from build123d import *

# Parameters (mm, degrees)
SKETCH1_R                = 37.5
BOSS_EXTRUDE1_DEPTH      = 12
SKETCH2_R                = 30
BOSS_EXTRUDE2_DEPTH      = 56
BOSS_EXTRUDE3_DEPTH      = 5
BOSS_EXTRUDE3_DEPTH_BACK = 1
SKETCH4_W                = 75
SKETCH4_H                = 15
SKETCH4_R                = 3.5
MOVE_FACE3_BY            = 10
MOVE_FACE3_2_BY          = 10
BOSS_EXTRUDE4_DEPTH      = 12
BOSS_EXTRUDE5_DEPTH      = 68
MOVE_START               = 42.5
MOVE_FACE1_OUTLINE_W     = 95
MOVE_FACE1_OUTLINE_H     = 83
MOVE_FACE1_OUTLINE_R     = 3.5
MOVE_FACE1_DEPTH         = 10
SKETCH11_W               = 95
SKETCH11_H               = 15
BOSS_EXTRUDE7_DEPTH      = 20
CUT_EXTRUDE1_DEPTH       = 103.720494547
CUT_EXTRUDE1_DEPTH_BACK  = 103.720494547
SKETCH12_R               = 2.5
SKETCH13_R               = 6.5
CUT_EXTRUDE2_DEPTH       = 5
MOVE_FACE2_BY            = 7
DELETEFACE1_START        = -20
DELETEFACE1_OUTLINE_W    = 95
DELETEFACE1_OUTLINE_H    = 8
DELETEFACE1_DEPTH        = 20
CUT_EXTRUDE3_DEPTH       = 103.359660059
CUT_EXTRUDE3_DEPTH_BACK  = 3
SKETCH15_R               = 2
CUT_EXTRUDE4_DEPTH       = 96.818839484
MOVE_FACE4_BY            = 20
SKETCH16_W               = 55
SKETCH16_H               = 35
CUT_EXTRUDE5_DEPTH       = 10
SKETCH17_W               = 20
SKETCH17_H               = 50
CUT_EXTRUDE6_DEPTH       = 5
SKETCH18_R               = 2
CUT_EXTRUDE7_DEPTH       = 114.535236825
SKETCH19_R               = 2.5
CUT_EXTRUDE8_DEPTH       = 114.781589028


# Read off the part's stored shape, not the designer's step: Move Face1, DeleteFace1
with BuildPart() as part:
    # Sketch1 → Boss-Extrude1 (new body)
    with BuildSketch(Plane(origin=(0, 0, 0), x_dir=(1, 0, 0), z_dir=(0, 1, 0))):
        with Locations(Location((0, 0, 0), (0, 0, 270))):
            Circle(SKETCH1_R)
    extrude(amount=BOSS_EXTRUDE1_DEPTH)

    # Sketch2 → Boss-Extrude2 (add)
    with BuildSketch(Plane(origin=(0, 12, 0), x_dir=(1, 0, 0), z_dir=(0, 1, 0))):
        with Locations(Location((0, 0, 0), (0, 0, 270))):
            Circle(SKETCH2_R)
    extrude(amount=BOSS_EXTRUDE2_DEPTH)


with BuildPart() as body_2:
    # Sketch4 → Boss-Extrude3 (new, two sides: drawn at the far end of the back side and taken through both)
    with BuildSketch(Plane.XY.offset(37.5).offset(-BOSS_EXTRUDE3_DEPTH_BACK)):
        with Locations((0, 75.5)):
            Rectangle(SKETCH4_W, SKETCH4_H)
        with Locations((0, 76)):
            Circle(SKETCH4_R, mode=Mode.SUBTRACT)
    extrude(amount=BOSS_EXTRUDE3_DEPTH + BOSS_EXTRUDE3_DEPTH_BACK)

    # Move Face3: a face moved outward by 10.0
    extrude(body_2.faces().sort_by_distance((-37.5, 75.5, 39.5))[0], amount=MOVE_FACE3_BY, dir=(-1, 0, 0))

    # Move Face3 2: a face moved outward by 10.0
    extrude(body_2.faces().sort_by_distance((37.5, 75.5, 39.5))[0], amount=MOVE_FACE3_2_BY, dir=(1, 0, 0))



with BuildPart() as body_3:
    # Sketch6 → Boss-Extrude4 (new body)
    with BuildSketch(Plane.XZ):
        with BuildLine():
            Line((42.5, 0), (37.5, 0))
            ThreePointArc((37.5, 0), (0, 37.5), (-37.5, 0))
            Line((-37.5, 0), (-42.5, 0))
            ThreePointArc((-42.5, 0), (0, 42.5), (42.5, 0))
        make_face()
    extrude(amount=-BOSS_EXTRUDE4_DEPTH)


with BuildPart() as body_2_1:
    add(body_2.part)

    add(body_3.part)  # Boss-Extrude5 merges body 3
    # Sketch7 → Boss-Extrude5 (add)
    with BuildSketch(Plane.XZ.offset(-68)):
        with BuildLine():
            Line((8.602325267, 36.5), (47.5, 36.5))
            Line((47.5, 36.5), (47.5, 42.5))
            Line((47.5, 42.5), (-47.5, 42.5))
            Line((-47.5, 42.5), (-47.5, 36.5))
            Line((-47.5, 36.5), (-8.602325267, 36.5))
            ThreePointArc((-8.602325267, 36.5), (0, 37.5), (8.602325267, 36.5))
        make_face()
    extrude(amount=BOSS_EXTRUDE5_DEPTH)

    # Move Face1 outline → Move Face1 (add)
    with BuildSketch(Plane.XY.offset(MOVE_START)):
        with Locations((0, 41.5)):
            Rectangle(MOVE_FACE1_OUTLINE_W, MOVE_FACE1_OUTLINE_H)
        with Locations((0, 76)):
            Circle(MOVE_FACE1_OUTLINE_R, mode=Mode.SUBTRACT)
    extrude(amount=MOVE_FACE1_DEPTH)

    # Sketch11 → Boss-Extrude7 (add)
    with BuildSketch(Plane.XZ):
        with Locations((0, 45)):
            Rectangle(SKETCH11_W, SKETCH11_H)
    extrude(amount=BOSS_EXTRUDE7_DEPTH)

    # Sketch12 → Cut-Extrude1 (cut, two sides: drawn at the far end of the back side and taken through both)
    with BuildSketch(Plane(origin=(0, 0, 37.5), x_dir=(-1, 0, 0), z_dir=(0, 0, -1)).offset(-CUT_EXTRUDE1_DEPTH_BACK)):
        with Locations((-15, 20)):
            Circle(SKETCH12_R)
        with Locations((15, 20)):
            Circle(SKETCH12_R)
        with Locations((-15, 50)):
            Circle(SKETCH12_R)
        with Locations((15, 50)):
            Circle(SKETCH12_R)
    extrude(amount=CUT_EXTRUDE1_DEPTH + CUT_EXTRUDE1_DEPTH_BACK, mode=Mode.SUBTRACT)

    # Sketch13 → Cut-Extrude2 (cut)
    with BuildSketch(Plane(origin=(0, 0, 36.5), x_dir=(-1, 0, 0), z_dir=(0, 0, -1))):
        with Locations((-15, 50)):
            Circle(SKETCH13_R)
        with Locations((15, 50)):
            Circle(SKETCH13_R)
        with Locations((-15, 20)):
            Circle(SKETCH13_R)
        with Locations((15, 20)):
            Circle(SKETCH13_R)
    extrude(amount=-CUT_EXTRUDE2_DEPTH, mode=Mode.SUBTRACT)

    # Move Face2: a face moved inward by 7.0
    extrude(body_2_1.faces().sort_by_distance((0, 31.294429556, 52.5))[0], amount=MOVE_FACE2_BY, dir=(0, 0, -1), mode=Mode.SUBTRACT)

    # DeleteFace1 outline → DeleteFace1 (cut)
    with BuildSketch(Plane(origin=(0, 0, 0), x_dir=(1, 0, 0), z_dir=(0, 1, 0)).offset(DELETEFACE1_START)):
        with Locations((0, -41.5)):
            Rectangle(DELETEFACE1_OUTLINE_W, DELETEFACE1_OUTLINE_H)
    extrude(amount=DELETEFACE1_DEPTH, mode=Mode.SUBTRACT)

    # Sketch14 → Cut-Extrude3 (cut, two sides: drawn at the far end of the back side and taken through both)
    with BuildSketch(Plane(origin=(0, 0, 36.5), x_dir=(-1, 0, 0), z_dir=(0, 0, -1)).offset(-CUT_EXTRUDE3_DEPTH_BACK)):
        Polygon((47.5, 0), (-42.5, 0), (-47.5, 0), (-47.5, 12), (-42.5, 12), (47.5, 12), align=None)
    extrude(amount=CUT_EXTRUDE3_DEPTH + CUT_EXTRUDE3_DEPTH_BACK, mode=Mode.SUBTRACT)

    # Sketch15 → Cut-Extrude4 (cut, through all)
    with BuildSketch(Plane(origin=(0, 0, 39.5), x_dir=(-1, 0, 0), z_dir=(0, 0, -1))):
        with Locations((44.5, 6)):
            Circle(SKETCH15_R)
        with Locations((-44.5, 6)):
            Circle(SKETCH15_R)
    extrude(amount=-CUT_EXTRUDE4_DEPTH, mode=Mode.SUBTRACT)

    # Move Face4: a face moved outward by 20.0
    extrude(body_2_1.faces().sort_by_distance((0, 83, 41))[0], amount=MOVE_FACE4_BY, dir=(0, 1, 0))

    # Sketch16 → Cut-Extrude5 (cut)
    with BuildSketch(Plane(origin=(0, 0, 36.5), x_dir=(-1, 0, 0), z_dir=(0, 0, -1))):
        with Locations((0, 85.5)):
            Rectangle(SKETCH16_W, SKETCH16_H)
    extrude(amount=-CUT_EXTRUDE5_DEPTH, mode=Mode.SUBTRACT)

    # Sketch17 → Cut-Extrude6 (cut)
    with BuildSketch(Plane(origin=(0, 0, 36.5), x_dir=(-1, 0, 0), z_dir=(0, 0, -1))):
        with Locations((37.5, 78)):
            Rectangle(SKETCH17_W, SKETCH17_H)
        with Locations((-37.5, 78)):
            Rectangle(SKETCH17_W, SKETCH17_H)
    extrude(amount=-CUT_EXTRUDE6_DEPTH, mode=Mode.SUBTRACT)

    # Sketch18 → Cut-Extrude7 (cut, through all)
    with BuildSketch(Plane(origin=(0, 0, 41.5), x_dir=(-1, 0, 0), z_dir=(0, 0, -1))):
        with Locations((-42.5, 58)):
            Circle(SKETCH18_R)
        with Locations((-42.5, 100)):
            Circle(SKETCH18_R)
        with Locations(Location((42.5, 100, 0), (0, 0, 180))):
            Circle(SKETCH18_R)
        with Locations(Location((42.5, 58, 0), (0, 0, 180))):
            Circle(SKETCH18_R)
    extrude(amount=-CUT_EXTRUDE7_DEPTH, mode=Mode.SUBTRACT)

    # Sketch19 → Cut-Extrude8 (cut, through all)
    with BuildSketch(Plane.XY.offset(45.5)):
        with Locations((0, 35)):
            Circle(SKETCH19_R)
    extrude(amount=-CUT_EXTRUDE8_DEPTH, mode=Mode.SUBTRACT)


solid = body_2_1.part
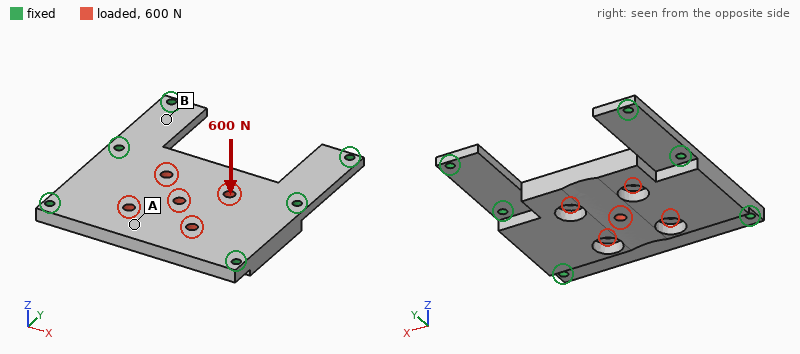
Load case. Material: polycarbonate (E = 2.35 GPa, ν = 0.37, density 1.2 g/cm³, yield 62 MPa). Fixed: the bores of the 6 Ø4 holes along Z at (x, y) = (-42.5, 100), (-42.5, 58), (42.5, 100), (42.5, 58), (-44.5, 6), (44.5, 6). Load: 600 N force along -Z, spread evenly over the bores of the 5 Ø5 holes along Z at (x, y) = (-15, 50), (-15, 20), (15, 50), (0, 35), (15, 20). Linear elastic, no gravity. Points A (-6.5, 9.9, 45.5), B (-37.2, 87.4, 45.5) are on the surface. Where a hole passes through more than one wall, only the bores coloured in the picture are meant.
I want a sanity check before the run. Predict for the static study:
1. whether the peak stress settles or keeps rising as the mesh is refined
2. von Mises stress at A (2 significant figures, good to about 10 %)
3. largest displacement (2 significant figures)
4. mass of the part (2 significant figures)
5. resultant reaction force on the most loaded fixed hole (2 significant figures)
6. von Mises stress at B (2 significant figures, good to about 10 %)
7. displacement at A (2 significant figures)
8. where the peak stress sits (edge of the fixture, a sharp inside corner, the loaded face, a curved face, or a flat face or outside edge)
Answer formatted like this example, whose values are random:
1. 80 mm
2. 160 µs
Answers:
1. keeps rising
2. 7.0 MPa
3. 0.65 mm
4. 64 g
5. 270 N
6. 2.8 MPa
7. 0.59 mm
8. edge of the fixture
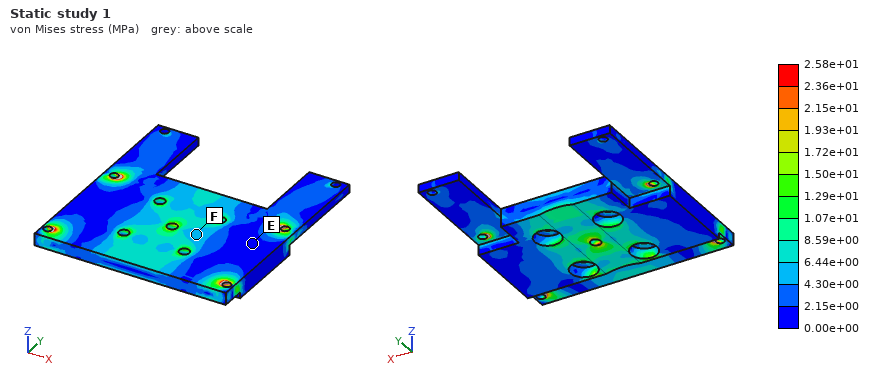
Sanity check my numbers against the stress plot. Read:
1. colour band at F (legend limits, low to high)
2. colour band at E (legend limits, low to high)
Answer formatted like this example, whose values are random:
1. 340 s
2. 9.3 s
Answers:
1. 4.30e+00 to 6.44e+00 MPa
2. 0.00e+00 to 2.15e+00 MPa
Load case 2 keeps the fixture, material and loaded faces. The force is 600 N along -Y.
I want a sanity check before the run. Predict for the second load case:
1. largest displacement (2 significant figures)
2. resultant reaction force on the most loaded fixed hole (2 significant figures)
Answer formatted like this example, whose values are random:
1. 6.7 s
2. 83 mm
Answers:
1. 52 µm
2. 170 N
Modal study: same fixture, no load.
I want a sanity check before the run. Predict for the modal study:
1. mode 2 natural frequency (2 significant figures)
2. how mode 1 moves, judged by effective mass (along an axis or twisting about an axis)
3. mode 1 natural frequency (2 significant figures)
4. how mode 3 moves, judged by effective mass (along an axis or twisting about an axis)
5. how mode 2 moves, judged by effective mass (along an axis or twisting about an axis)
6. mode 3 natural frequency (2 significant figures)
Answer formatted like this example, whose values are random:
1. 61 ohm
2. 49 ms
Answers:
1. 1500 Hz
2. along Z
3. 950 Hz
4. twisting about Y
5. twisting about X
6. 2500 Hz
